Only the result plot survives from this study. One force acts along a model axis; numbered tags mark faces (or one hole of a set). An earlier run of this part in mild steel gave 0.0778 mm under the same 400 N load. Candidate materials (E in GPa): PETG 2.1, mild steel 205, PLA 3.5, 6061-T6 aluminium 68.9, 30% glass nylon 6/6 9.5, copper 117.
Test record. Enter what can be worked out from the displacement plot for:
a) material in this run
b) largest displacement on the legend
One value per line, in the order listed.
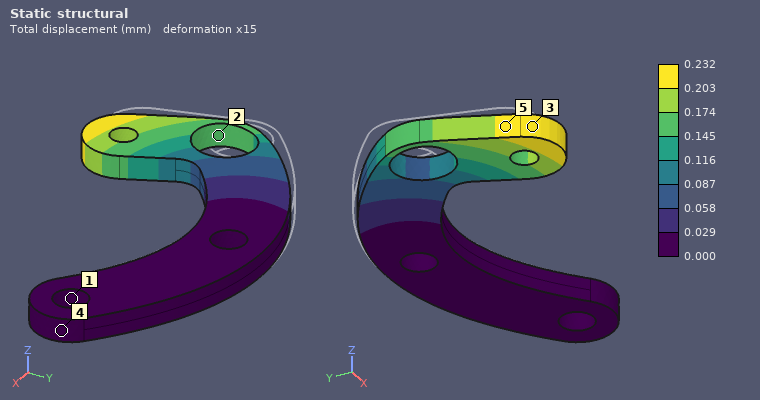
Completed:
6061-T6 aluminium
0.232 mm
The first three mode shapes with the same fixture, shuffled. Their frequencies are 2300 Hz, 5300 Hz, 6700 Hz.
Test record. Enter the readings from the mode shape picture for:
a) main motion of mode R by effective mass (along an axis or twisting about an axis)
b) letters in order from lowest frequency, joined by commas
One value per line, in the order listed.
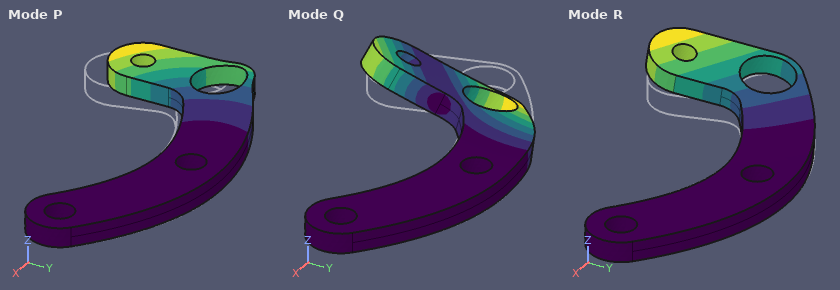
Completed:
along Z
R, P, Q
